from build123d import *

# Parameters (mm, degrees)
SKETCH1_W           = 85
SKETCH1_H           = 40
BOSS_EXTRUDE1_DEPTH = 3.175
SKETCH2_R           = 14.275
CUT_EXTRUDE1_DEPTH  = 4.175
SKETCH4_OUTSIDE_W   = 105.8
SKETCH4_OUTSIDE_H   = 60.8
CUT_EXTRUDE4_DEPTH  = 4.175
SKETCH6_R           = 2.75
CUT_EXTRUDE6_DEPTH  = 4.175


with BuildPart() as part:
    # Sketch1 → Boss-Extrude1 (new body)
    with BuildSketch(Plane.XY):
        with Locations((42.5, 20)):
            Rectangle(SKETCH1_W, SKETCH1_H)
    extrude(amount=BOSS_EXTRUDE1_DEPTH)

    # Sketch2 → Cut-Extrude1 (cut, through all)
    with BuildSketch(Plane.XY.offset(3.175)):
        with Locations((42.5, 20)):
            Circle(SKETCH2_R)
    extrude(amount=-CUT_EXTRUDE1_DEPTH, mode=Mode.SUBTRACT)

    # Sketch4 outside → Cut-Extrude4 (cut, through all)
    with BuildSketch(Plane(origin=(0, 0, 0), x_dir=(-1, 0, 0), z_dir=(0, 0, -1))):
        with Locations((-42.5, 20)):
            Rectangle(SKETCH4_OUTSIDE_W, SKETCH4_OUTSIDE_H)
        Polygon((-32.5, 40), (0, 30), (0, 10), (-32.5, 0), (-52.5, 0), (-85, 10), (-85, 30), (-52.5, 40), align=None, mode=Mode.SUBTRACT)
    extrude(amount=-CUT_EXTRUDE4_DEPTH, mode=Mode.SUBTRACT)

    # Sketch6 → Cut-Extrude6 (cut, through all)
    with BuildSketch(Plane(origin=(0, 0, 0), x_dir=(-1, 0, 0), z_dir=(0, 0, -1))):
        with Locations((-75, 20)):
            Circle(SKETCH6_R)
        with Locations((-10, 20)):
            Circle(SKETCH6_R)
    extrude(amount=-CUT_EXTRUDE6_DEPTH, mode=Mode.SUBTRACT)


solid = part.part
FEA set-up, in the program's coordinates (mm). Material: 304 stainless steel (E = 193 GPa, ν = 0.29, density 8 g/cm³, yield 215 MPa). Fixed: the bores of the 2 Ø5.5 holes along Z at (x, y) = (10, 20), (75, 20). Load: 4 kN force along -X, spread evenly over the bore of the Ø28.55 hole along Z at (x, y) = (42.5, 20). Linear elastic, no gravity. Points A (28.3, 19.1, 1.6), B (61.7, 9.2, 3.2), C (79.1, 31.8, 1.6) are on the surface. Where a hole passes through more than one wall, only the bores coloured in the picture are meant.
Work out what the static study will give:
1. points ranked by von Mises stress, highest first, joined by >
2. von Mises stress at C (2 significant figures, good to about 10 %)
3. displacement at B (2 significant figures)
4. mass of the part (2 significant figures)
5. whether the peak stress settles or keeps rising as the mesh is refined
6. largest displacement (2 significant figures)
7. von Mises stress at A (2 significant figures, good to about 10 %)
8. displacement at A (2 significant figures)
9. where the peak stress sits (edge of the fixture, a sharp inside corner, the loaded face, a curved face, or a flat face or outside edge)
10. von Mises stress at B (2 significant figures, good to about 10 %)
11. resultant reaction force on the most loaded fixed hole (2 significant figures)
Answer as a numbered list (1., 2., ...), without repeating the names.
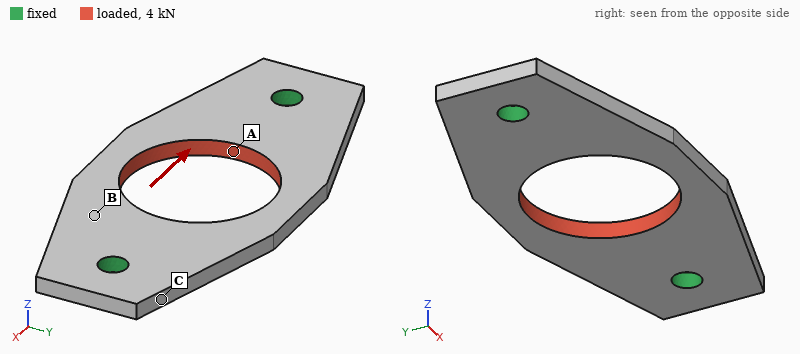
1. A > B > C
2. 11 MPa
3. 2.9 µm
4. 52 g
5. keeps rising
6. 5.4 µm
7. 38 MPa
8. 2.3 µm
9. edge of the fixture
10. 23 MPa
11. 2.0 kN
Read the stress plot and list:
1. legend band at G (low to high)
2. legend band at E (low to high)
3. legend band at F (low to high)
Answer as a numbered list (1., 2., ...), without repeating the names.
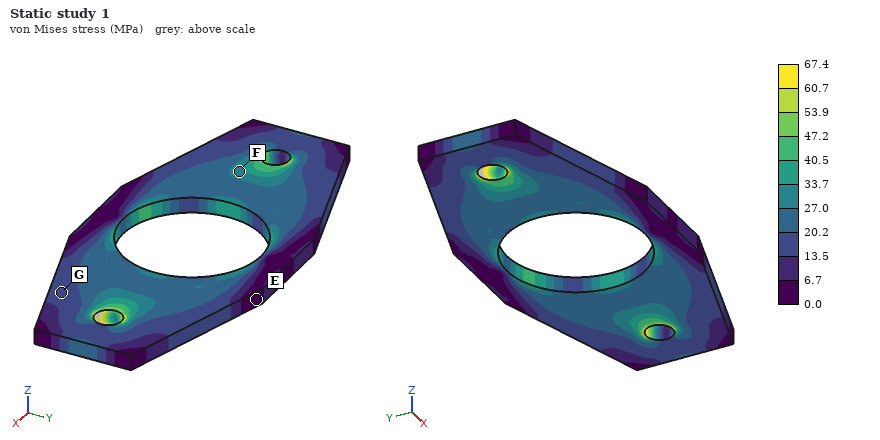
1. 13.5 to 20.2 MPa
2. 0.0 to 6.7 MPa
3. 27.0 to 33.7 MPa
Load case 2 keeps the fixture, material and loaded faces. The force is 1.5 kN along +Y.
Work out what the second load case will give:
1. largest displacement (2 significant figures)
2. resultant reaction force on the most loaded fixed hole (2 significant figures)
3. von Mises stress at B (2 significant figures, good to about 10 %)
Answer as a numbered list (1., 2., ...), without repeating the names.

1. 5.5 µm
2. 750 N
3. 13 MPa
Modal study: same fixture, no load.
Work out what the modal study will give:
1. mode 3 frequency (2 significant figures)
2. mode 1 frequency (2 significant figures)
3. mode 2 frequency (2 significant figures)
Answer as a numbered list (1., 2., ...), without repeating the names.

1. 8200 Hz
2. 3700 Hz
3. 3800 Hz
